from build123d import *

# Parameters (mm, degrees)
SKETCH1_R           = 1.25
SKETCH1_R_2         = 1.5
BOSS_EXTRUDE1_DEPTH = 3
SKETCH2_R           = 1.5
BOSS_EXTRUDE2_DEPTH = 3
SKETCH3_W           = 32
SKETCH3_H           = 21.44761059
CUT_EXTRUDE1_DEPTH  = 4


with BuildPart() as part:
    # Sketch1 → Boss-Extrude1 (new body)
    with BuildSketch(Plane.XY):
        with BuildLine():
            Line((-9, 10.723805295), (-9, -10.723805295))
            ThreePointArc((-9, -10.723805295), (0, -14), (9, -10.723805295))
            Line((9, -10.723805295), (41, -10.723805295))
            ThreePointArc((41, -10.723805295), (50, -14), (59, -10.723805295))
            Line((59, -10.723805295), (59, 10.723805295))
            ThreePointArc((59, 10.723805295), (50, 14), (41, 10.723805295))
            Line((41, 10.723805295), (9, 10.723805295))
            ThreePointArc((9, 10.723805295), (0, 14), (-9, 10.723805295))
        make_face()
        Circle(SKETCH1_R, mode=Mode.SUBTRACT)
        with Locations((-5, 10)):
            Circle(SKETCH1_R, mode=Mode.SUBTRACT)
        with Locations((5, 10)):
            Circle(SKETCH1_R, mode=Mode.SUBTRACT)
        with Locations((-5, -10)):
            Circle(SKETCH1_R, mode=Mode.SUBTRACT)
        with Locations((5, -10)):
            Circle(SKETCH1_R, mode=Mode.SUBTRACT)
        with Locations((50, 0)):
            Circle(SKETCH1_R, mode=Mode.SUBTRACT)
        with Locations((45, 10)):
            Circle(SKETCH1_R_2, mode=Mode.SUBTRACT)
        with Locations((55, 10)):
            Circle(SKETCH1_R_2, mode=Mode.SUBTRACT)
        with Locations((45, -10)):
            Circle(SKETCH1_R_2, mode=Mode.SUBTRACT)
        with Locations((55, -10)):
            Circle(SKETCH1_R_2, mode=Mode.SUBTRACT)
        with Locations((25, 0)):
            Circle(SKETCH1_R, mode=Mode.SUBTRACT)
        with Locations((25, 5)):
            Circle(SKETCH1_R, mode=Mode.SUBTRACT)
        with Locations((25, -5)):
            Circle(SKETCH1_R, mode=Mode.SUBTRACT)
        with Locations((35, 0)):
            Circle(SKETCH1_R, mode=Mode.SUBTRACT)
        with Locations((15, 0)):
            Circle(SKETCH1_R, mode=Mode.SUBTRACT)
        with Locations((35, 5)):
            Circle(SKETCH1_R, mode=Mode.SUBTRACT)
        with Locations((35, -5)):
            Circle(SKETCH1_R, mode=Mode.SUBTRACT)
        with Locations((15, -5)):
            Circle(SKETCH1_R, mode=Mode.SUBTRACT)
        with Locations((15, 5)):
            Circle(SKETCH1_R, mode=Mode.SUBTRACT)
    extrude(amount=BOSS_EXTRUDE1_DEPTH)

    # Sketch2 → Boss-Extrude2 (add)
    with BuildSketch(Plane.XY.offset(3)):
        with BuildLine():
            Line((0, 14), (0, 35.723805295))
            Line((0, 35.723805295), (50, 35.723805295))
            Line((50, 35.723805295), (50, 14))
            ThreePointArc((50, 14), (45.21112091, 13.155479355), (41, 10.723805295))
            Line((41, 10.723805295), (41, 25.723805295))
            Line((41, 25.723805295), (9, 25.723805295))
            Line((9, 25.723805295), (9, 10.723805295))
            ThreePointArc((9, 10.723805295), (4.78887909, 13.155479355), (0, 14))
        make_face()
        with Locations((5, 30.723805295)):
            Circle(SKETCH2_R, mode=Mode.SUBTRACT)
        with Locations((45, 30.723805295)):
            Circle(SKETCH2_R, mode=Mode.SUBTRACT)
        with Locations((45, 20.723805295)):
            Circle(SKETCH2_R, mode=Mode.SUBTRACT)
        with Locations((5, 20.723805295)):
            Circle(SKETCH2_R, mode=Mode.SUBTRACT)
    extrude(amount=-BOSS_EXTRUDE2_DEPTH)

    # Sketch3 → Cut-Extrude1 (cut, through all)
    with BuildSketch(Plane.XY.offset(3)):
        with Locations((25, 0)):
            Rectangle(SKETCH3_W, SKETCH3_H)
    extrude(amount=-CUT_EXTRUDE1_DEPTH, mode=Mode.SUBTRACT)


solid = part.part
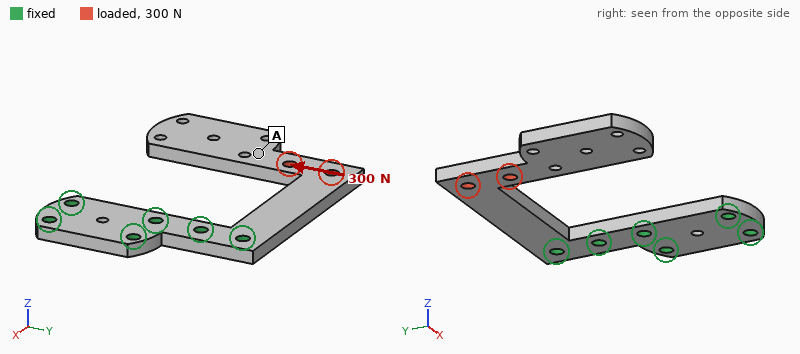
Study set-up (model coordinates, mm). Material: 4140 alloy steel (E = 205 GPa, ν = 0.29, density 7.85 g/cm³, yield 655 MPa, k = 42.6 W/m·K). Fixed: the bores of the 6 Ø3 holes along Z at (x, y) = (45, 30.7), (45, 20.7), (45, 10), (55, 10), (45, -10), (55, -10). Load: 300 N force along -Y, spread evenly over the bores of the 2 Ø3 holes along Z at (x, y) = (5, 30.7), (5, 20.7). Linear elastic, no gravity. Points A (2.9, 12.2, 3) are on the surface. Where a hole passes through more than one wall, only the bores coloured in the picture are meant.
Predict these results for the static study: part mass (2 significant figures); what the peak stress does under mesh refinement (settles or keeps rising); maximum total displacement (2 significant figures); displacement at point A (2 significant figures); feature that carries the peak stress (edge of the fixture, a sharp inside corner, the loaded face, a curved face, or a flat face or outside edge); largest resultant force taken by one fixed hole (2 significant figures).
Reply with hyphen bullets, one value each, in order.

- 37 g
- keeps rising
- 0.29 mm
- 0.17 mm
- edge of the fixture
- 960 N
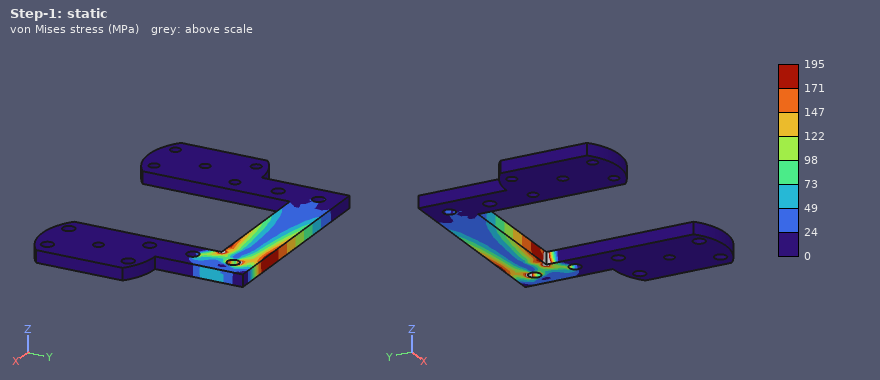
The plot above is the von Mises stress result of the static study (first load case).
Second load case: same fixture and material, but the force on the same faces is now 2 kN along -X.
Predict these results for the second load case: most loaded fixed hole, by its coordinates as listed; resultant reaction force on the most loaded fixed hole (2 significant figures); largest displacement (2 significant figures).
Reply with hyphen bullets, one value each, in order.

- (45, 30.7)
- 1.2 kN
- 0.46 mm
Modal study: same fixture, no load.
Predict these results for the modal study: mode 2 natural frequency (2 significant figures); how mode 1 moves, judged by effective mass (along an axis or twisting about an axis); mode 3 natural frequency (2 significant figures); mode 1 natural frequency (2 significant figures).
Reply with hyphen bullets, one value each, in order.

- 1100 Hz
- along Z
- 1300 Hz
- 380 Hz
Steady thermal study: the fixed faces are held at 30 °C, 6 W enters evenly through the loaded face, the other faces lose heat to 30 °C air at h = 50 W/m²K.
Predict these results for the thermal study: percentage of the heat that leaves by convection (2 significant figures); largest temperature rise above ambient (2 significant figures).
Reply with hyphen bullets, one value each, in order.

- 74 %
- 63 K
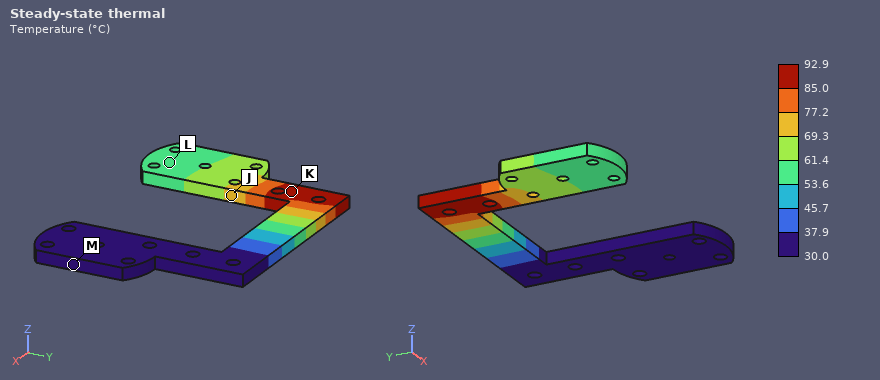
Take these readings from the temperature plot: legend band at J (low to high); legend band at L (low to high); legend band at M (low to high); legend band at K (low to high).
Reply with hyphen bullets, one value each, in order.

- 69.3 to 77.2 °C
- 53.6 to 61.4 °C
- 30.0 to 37.9 °C
- 85.0 to 92.9 °C
